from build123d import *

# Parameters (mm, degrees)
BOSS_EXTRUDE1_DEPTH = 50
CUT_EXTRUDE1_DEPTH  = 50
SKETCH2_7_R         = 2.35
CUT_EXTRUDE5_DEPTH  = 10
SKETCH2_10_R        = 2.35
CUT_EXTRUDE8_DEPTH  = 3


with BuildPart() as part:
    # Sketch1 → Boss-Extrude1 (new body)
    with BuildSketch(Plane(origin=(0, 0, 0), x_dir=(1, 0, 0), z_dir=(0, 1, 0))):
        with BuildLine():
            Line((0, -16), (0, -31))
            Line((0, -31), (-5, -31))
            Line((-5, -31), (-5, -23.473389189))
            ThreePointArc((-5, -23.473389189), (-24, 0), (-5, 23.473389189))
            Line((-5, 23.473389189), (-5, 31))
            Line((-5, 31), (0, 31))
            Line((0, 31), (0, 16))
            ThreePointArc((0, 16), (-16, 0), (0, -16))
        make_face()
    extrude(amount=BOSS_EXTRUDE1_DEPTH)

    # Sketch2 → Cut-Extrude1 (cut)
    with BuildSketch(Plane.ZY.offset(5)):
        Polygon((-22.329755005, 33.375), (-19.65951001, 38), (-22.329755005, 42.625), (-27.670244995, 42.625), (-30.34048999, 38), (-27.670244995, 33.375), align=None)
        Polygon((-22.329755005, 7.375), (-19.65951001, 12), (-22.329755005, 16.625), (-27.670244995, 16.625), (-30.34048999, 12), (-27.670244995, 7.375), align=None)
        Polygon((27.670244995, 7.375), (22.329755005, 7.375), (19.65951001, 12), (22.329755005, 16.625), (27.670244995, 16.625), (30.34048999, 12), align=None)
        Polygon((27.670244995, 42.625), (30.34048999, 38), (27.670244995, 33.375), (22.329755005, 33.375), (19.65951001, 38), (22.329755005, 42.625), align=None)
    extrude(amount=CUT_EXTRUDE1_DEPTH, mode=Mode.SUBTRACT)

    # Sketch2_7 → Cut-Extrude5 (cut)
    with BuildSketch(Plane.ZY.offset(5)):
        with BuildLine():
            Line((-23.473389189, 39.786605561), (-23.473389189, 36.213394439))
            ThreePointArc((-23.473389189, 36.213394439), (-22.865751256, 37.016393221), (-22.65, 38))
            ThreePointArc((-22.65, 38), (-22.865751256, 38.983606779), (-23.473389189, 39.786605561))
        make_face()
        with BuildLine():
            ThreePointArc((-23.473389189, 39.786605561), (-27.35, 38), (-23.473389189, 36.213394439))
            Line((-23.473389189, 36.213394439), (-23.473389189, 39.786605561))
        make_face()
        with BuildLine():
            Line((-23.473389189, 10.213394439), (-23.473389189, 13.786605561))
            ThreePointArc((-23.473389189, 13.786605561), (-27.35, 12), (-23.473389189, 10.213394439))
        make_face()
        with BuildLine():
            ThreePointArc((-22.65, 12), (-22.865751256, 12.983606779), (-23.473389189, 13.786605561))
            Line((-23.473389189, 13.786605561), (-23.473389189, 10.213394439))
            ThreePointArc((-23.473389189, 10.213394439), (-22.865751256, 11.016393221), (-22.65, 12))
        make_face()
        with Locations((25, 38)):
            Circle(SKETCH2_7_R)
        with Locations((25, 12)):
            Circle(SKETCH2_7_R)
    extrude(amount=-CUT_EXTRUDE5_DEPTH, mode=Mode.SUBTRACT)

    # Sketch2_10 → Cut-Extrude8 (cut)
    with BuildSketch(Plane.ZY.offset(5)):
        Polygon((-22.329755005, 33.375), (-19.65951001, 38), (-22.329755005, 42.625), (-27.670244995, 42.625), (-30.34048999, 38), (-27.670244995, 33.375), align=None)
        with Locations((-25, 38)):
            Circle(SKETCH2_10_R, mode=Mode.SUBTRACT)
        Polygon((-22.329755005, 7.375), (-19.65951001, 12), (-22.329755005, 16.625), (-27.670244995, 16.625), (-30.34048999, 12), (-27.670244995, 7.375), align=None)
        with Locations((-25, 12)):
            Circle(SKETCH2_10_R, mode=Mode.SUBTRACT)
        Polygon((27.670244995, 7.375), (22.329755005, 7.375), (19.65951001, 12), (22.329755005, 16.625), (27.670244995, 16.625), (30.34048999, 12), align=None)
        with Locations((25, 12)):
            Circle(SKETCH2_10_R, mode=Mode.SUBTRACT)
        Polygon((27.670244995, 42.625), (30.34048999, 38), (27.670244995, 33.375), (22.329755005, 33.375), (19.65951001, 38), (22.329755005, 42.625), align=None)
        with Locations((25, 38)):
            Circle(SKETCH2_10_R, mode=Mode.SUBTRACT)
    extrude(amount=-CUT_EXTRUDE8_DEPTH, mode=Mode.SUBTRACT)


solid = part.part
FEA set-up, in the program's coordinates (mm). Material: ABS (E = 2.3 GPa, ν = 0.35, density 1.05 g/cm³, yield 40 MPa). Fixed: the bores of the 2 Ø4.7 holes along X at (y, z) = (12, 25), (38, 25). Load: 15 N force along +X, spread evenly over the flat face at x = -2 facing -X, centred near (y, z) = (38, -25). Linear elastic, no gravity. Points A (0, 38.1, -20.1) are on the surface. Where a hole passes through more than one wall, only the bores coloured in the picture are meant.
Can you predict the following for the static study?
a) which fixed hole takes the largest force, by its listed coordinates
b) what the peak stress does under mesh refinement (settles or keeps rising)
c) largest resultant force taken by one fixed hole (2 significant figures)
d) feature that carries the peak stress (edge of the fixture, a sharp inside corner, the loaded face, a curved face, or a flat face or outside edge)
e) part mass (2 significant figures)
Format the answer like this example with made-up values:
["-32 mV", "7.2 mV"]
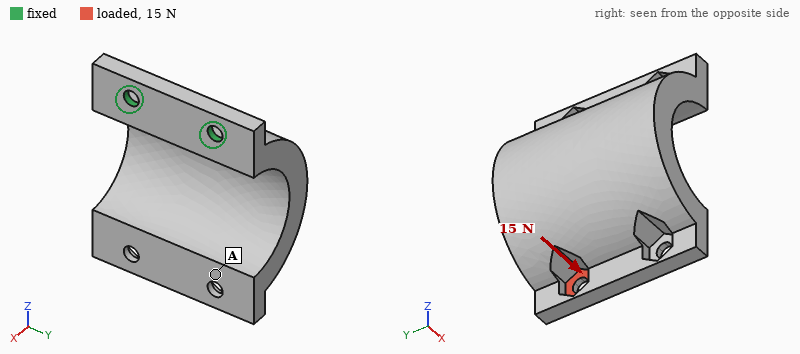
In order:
["(38, 25)", "keeps rising", "15 N", "edge of the fixture", "29 g"]
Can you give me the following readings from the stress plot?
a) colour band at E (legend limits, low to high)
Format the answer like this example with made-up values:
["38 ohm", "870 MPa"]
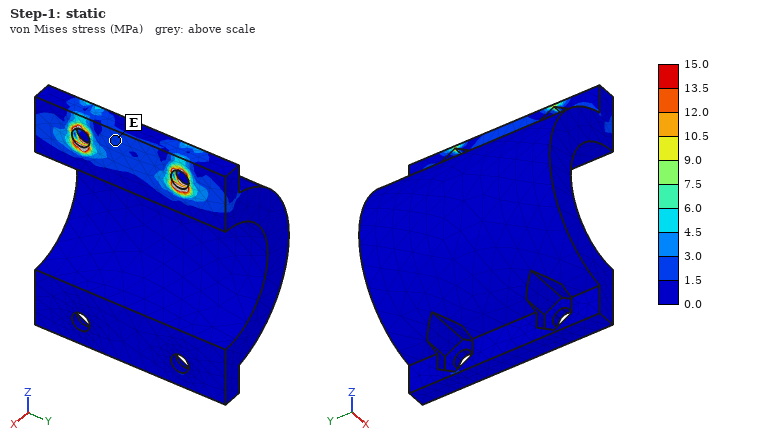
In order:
["1.5 to 3.0 MPa"]
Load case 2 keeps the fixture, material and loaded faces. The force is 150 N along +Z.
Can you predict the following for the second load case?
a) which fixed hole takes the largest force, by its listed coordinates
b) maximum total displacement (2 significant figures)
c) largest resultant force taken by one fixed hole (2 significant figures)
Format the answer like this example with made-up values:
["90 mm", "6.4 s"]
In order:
["(38, 25)", "0.75 mm", "140 N"]
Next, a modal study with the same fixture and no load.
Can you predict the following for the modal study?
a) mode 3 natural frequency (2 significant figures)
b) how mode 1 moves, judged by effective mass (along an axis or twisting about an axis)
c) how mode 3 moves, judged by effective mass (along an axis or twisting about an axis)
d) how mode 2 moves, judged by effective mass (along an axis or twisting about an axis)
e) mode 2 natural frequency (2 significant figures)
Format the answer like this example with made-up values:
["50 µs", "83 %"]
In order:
["1200 Hz", "along X", "along Z", "along Y", "650 Hz"]
